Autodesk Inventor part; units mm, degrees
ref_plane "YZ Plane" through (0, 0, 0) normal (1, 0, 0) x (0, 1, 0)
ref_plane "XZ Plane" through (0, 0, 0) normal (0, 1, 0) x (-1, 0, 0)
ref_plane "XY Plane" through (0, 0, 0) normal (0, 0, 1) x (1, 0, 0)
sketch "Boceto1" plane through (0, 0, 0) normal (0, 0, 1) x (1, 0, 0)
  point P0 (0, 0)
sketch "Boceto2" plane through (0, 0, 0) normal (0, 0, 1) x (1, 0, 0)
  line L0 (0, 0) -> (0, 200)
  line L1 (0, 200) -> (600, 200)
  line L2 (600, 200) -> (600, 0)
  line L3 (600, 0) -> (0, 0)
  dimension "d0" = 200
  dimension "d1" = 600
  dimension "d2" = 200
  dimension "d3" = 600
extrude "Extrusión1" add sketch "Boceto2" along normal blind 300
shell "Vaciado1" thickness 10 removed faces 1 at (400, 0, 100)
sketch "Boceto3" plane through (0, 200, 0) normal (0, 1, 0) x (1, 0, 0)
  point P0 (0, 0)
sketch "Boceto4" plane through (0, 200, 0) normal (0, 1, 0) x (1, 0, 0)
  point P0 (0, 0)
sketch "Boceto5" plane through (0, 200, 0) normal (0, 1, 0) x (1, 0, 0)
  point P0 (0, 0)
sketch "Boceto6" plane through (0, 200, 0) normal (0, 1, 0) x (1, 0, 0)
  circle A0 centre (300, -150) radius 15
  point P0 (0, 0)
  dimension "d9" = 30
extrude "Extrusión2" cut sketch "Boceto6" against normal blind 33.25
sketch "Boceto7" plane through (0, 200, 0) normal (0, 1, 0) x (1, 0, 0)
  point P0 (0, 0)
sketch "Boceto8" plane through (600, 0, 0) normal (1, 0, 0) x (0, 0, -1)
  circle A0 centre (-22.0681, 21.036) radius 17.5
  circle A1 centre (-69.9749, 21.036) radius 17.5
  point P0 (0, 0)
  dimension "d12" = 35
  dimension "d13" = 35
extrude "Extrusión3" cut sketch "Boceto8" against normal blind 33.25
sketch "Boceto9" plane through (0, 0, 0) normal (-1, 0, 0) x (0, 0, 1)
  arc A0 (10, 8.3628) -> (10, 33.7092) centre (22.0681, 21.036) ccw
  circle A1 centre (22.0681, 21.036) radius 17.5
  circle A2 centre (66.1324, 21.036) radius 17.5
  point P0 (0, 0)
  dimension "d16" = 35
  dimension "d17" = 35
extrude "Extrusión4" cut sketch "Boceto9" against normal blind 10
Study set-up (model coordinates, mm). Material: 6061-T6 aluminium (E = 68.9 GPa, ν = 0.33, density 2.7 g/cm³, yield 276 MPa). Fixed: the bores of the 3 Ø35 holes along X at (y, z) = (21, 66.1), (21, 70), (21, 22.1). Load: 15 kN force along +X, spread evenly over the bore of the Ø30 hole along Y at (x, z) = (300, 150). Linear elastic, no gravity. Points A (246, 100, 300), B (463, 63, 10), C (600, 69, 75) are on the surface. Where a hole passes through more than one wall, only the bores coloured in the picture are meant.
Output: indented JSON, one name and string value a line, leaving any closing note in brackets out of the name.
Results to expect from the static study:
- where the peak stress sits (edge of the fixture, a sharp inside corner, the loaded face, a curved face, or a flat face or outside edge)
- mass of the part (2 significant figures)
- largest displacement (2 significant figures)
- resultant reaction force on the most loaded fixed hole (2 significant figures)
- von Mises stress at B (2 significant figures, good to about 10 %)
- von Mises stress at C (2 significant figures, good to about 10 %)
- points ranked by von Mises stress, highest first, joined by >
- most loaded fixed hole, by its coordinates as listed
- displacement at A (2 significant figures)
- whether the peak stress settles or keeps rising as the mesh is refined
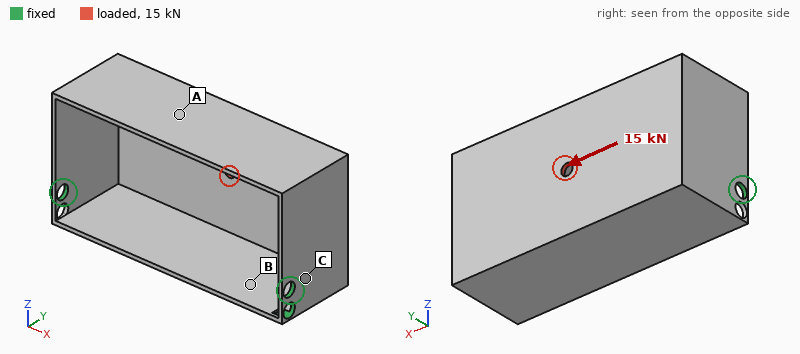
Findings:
{
  "where the peak stress sits": "a sharp inside corner",
  "mass of the part": "14 kg",
  "largest displacement": "0.51 mm",
  "resultant reaction force on the most loaded fixed hole": "17 kN",
  "von Mises stress at B": "10 MPa",
  "von Mises stress at C": "15 MPa",
  "points ranked by von Mises stress, highest first, joined by >": "C > B > A",
  "most loaded fixed hole, by its coordinates as listed": "(21, 22.1)",
  "displacement at A": "0.35 mm",
  "whether the peak stress settles or keeps rising as the mesh is refined": "keeps rising"
}
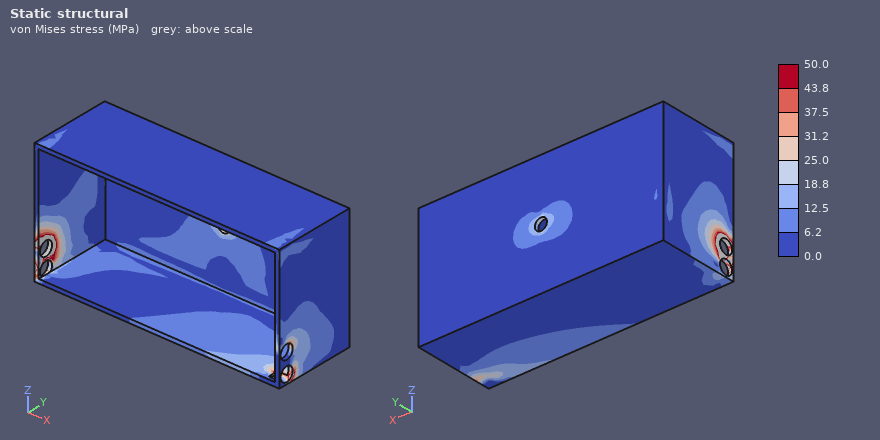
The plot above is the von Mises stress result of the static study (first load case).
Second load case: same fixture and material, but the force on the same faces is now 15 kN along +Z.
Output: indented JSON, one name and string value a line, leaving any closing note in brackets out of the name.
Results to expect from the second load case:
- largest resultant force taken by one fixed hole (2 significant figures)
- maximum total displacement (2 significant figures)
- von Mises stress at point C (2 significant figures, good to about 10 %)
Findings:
{
  "largest resultant force taken by one fixed hole": "17 kN",
  "maximum total displacement": "0.65 mm",
  "von Mises stress at point C": "21 MPa"
}
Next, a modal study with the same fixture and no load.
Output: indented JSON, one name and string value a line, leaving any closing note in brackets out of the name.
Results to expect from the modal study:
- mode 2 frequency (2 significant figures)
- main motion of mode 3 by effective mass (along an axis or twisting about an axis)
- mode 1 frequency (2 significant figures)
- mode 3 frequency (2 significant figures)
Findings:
{
  "mode 2 frequency": "240 Hz",
  "main motion of mode 3 by effective mass": "along Z",
  "mode 1 frequency": "230 Hz",
  "mode 3 frequency": "270 Hz"
}
